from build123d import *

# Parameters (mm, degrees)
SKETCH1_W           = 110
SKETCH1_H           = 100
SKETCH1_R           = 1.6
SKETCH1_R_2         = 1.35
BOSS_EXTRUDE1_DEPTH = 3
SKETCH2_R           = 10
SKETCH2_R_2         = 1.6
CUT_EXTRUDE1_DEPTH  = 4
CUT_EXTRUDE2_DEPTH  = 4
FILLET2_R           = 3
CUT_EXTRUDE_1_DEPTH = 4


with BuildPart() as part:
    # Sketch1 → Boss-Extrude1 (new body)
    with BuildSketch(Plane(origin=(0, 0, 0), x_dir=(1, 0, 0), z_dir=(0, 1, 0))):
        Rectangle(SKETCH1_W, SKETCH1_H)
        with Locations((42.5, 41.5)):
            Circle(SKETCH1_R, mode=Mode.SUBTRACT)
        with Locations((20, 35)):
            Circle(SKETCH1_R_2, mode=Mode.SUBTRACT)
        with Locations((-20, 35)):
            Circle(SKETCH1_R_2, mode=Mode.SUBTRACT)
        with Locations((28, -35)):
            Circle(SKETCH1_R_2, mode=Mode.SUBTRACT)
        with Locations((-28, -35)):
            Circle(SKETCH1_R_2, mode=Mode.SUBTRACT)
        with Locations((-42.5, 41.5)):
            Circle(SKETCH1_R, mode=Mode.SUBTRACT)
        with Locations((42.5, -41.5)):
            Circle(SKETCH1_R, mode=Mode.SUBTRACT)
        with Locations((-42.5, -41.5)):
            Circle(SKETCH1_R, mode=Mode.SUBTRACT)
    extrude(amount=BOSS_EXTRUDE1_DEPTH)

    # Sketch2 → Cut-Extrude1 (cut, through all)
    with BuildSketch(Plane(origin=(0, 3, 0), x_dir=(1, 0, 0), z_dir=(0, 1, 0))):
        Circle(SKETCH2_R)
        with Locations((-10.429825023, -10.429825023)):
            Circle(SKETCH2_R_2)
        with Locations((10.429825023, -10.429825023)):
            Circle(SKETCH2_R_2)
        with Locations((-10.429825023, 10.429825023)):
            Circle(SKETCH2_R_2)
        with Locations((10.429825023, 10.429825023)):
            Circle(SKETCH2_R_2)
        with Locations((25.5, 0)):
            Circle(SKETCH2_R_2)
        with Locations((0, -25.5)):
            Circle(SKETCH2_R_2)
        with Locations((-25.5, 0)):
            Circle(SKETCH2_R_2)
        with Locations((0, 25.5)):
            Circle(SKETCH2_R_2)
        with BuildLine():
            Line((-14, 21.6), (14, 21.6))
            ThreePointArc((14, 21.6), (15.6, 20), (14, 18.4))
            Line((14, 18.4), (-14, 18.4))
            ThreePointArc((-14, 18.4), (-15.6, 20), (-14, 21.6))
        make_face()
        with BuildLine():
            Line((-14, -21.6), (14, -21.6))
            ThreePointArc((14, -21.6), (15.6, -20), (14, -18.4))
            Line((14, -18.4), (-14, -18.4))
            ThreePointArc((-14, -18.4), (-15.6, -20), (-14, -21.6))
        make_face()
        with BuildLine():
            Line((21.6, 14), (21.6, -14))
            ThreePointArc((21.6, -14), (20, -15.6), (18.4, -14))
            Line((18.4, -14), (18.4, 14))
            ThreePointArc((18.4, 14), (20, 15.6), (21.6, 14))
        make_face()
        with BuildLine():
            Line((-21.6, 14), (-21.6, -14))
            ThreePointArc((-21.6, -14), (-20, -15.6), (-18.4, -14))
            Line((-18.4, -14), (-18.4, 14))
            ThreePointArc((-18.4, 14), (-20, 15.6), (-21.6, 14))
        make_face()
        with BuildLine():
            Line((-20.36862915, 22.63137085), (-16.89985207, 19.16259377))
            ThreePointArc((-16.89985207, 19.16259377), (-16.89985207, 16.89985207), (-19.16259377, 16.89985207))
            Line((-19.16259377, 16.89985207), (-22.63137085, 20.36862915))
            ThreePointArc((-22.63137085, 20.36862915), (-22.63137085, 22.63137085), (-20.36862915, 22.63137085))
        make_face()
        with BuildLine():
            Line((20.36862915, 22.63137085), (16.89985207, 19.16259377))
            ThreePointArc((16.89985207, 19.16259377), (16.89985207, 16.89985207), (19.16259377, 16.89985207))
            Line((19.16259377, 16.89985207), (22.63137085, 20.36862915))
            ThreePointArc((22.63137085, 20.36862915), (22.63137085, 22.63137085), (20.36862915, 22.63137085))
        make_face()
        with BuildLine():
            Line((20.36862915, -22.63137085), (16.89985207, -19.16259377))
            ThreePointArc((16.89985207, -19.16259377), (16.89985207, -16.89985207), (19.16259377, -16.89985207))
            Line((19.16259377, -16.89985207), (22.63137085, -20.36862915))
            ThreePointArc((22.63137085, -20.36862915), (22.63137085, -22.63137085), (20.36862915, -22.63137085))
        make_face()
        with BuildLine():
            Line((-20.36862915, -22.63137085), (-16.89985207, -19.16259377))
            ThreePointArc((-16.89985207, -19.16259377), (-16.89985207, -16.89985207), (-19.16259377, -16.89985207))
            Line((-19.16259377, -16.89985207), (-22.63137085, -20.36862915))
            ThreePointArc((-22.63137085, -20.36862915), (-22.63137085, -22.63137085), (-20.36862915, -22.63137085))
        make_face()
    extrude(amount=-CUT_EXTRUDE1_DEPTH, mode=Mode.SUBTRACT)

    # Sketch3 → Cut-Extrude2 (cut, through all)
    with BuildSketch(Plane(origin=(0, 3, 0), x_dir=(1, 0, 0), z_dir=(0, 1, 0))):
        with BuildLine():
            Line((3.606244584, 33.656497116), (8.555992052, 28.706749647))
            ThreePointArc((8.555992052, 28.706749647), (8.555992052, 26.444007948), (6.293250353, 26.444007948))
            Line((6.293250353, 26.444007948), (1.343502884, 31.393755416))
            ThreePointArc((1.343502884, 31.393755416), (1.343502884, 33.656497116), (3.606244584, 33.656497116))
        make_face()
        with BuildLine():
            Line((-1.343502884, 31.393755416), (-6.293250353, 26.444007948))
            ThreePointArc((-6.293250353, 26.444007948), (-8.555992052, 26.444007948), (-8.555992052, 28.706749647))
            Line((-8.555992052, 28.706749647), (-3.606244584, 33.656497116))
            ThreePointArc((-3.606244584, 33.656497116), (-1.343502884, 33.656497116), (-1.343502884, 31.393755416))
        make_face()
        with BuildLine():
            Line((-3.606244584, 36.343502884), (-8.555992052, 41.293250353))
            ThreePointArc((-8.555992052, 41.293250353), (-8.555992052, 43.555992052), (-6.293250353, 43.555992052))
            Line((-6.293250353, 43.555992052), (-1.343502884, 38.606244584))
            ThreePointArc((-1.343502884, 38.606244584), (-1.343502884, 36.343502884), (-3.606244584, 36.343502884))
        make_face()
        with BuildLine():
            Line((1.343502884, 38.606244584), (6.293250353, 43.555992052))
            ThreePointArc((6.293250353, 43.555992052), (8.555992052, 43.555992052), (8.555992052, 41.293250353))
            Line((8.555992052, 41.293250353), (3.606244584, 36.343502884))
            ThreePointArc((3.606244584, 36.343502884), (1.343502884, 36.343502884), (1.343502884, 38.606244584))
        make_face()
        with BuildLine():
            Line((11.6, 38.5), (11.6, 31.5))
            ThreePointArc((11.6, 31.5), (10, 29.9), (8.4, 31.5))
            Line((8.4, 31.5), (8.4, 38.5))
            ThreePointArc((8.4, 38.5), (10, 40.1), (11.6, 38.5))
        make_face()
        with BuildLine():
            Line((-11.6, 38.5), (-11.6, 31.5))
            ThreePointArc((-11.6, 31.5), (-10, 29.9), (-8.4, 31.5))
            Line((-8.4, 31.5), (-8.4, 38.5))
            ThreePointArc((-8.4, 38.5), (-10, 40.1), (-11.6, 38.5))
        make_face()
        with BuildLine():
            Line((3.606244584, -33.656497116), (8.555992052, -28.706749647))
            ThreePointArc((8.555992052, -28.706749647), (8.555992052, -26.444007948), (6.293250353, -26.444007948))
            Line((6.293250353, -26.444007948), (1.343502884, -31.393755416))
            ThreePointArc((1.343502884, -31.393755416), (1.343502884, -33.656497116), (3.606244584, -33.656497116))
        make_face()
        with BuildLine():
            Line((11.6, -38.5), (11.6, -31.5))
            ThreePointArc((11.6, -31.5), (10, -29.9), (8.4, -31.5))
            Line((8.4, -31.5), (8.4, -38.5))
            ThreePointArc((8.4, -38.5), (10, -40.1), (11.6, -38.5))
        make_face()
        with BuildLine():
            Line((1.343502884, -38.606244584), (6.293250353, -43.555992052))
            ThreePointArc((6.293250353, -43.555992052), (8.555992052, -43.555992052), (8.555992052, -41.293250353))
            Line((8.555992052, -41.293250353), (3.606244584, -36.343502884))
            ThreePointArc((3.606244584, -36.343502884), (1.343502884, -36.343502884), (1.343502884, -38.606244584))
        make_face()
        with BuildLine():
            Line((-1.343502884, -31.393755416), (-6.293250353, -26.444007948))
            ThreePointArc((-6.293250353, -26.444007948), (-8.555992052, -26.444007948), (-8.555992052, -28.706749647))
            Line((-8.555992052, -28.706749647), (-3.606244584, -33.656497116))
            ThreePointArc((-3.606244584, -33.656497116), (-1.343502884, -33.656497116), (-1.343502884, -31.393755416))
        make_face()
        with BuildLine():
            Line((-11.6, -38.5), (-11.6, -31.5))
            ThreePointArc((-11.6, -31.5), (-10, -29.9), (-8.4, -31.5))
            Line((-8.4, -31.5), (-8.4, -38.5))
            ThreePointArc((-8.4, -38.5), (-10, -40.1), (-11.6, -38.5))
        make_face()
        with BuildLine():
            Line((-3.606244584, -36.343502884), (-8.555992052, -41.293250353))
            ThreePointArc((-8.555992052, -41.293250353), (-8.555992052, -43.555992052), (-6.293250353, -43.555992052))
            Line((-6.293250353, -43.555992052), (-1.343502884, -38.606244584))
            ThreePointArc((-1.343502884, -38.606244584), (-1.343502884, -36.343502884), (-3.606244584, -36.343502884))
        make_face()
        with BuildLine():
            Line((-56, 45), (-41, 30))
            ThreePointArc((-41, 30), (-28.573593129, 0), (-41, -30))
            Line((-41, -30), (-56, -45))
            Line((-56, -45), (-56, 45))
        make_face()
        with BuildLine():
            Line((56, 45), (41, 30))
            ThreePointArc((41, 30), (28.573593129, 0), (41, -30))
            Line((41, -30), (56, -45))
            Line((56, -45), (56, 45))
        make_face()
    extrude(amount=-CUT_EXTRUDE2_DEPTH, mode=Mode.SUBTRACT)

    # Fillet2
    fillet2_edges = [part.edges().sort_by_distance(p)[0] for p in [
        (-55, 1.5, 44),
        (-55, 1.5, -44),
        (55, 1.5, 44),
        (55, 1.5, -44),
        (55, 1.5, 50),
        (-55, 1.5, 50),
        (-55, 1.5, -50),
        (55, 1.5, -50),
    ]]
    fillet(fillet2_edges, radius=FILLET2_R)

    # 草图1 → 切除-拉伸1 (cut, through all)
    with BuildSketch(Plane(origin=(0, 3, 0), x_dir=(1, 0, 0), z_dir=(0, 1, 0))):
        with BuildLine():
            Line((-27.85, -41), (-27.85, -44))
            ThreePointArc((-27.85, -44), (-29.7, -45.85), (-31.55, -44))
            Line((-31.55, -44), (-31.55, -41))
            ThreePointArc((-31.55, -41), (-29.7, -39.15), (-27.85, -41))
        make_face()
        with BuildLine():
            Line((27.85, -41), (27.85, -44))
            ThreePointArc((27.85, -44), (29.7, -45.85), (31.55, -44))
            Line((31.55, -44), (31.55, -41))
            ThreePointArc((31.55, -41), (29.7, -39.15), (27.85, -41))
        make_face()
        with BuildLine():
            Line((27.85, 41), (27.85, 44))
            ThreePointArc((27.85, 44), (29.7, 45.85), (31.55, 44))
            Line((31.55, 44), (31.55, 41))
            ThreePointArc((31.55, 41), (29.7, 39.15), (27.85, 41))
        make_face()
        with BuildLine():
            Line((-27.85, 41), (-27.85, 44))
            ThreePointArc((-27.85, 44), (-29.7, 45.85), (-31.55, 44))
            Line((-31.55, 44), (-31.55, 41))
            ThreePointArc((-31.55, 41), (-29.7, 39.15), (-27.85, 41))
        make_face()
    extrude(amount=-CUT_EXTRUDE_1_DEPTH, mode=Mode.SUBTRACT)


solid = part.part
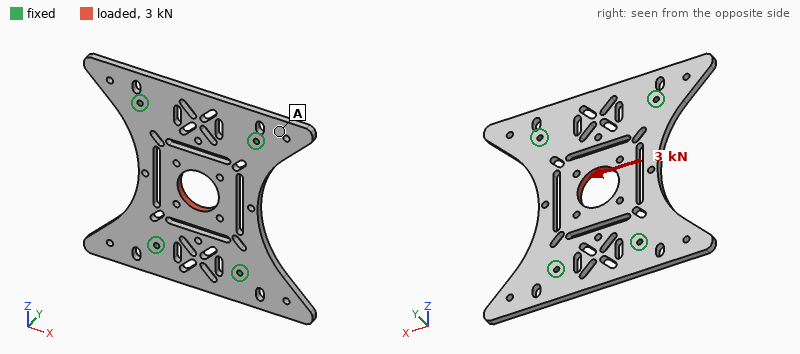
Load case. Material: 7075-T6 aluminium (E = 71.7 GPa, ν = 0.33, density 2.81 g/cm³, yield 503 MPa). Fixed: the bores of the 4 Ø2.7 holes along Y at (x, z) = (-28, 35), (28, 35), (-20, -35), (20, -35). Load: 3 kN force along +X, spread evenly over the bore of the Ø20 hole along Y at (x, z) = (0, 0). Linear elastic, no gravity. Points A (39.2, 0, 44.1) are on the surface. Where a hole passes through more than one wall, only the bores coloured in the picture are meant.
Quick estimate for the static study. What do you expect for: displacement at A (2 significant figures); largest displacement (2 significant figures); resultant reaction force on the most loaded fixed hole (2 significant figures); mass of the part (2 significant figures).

7.3 µm
41 µm
1.0 kN
55 g
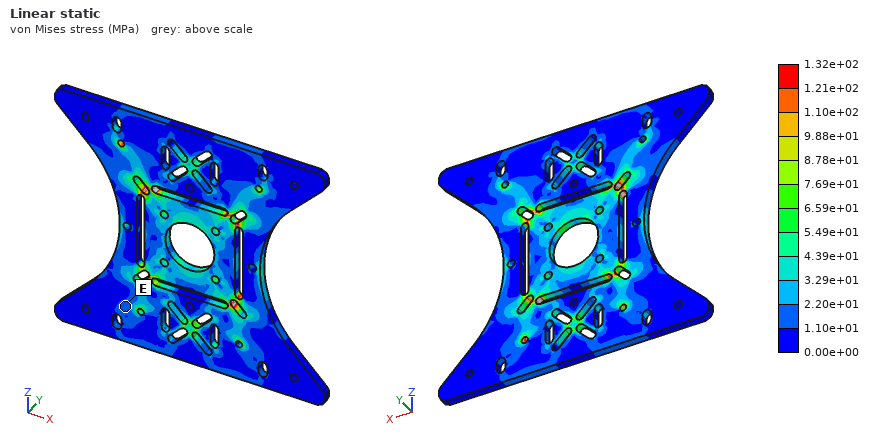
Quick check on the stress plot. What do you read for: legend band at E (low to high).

1.10e+01 to 2.20e+01 MPa
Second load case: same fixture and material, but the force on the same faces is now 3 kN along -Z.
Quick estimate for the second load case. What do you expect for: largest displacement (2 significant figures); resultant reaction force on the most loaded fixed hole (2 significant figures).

29 µm
810 N
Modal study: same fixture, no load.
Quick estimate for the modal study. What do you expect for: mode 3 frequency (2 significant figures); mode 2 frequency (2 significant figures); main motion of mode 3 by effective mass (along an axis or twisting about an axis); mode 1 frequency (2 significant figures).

2700 Hz
2500 Hz
along Y
2400 Hz
